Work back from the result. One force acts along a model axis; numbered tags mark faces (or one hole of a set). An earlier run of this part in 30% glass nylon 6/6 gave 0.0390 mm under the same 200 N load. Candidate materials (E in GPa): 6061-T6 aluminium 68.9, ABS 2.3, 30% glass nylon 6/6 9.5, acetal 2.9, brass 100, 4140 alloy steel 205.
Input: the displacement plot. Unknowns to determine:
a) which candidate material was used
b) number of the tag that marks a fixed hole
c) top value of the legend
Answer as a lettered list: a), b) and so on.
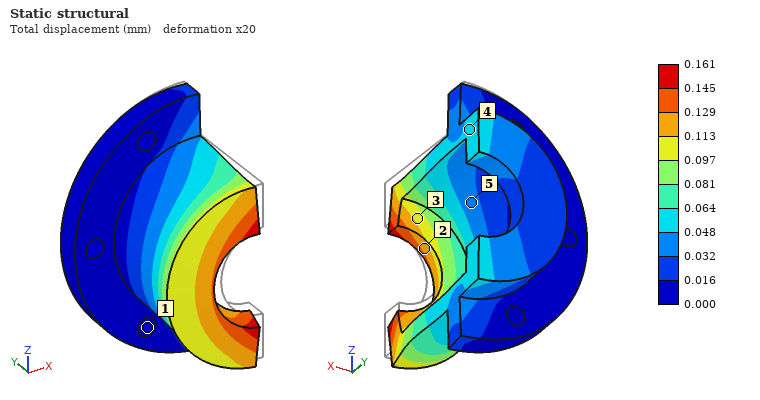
a) ABS
b) 1
c) 0.161 mm
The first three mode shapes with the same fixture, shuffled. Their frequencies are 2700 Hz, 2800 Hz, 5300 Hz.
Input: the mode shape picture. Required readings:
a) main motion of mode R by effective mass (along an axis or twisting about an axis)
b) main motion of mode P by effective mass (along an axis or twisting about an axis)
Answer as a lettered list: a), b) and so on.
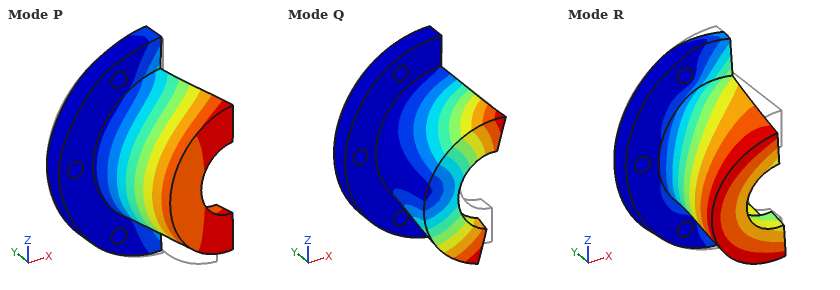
a) along Z
b) along X
